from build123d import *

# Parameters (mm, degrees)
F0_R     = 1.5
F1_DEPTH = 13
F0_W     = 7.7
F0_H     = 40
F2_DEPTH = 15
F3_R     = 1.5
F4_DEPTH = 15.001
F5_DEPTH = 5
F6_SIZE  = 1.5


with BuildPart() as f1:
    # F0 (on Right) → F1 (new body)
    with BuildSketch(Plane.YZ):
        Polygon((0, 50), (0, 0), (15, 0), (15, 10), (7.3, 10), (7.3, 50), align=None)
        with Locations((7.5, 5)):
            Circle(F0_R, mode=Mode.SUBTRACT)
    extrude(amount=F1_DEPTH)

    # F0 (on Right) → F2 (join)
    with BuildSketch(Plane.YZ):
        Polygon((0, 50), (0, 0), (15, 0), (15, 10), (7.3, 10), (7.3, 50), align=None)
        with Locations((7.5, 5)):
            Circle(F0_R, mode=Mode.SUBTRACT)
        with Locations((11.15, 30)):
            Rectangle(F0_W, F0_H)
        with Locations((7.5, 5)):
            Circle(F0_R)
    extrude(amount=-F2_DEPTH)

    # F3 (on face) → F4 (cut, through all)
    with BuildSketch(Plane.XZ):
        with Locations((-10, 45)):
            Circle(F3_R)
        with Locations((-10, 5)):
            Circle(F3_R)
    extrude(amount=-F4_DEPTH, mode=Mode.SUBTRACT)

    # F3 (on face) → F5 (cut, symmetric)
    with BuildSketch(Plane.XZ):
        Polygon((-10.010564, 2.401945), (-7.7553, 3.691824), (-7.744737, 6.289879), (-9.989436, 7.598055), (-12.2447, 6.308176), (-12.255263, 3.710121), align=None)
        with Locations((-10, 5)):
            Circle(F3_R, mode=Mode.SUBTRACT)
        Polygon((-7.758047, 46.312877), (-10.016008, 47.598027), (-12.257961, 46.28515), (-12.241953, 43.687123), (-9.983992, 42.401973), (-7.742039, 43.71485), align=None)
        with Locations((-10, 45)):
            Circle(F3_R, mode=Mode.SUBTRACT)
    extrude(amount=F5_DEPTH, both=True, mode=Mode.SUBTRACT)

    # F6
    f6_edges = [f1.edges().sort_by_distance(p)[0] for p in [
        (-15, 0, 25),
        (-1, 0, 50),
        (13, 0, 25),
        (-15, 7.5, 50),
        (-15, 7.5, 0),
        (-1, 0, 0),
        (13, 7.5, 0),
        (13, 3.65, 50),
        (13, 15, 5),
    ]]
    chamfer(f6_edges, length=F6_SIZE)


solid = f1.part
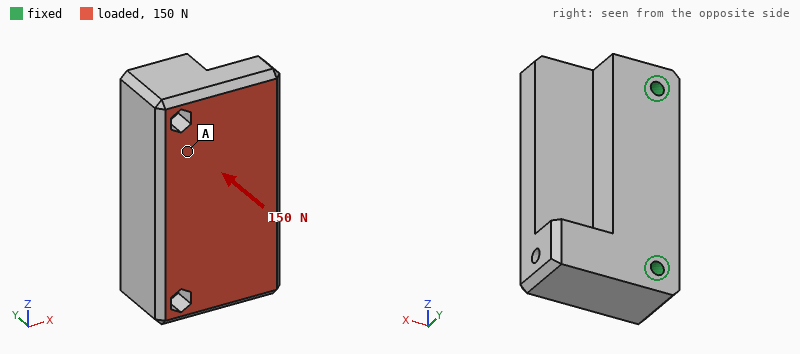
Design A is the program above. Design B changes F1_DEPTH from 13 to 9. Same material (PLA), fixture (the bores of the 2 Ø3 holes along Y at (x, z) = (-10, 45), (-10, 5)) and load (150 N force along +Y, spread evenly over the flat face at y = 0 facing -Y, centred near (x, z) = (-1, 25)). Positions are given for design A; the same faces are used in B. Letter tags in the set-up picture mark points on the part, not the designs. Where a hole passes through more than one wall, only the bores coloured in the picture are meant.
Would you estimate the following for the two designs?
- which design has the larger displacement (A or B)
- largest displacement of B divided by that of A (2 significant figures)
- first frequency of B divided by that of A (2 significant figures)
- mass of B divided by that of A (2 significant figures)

A
0.68
1.3
0.89
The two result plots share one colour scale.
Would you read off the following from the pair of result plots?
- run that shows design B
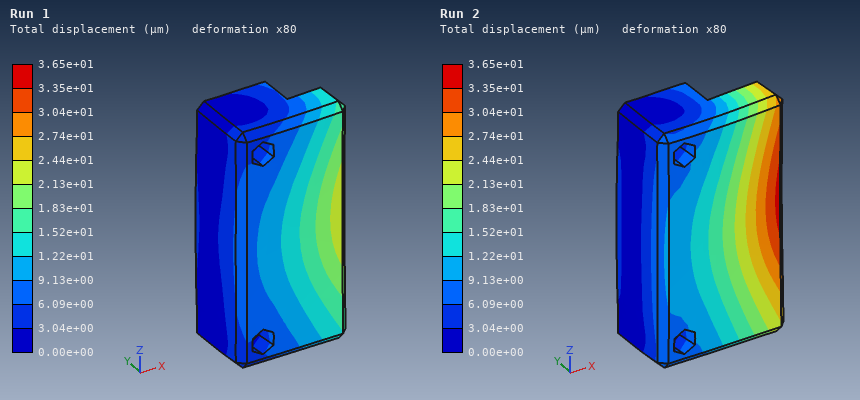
Run 1
